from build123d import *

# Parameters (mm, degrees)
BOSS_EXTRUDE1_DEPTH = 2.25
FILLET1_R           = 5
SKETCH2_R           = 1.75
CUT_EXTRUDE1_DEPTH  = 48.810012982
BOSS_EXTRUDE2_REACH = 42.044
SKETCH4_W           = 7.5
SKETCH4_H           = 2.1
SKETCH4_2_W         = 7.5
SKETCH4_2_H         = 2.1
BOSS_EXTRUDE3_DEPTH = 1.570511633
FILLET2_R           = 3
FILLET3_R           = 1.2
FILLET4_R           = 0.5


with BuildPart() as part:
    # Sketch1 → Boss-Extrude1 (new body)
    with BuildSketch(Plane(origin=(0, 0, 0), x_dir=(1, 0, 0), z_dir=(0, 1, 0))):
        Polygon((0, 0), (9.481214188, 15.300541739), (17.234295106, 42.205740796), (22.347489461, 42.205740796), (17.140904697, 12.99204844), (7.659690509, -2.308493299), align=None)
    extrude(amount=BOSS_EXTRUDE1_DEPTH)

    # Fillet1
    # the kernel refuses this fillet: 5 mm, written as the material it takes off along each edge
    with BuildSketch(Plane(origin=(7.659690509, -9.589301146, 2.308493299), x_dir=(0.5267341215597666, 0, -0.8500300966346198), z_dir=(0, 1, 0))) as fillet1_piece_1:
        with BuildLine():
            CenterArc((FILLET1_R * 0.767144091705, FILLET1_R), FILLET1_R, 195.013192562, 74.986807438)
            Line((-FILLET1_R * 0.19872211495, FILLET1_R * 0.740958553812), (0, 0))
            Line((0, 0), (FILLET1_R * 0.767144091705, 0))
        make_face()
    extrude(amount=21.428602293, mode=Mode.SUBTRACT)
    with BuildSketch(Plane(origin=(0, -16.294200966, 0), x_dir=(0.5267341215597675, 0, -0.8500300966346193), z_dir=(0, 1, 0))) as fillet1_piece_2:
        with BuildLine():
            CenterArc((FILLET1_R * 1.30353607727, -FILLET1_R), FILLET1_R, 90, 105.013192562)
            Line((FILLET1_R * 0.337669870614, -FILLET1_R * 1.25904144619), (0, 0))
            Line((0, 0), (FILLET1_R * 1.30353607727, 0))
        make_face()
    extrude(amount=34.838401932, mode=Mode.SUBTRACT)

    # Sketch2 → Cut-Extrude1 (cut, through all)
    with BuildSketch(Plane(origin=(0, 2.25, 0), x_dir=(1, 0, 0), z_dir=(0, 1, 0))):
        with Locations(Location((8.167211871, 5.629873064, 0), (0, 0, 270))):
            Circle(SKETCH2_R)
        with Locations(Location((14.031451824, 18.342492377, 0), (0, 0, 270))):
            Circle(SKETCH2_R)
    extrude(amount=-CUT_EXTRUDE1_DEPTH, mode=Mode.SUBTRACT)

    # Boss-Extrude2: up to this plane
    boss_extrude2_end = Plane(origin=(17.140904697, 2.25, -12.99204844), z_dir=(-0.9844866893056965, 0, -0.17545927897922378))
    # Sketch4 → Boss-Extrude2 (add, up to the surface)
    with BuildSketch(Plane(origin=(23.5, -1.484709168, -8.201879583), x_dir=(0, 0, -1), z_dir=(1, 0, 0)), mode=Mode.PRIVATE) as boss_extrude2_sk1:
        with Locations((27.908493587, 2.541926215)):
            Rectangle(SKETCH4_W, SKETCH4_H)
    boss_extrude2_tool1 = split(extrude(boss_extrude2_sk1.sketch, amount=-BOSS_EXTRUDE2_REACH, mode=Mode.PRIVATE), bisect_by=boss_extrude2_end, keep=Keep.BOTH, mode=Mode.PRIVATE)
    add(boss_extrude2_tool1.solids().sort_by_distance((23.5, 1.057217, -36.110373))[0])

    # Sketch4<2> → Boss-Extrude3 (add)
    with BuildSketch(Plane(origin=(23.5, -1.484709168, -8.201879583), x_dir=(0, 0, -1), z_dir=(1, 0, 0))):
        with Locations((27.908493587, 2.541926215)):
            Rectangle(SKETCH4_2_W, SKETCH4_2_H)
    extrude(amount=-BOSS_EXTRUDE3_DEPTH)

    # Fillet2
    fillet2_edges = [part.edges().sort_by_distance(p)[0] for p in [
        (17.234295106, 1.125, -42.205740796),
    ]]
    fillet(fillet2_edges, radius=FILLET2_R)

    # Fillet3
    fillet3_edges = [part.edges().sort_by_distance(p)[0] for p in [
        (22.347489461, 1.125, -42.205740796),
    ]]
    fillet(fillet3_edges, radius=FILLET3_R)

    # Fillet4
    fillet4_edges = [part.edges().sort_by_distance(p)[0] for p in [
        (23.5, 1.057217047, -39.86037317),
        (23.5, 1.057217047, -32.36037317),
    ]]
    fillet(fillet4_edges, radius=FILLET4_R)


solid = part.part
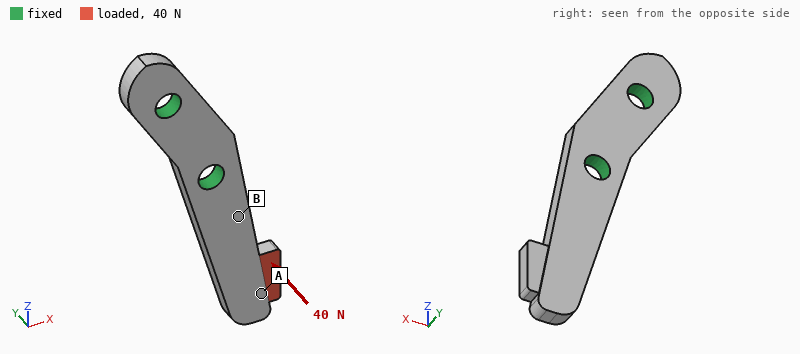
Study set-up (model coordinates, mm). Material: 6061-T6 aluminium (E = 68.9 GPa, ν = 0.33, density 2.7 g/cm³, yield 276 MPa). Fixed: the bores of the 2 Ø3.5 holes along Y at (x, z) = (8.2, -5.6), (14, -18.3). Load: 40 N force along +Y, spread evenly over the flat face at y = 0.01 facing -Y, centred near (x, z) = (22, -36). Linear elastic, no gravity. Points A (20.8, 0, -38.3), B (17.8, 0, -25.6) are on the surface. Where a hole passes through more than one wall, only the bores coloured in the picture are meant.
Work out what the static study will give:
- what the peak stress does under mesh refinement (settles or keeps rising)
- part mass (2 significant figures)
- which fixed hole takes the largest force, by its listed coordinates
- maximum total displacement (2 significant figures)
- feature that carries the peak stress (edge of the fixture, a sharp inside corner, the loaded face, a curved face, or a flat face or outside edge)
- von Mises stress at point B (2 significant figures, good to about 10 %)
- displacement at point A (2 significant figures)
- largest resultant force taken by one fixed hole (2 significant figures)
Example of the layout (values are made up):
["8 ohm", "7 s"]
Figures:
["keeps rising", "1.9 g", "(14, -18.3)", "0.25 mm", "edge of the fixture", "82 MPa", "0.20 mm", "40 N"]
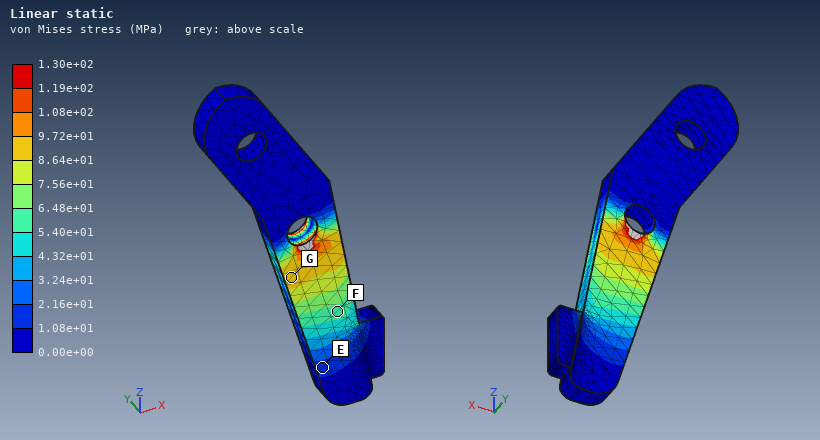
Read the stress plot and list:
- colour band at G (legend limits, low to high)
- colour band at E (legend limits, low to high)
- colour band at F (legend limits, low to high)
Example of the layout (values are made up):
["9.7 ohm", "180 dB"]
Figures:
["8.64e+01 to 9.72e+01 MPa", "1.08e+01 to 2.16e+01 MPa", "5.40e+01 to 6.48e+01 MPa"]
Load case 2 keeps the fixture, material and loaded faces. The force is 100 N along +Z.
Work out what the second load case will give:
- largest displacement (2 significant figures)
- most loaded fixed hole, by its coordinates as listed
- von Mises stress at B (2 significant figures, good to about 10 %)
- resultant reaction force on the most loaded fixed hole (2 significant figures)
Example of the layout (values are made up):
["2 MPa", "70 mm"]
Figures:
["81 µm", "(14, -18.3)", "46 MPa", "98 N"]
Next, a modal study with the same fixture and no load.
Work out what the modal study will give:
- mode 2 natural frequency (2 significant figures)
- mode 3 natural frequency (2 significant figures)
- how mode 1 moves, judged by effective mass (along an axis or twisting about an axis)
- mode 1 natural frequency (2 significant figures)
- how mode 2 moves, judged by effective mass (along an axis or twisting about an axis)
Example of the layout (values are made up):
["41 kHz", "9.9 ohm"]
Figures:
["9000 Hz", "18 kHz", "along Y", "3500 Hz", "along X"]
